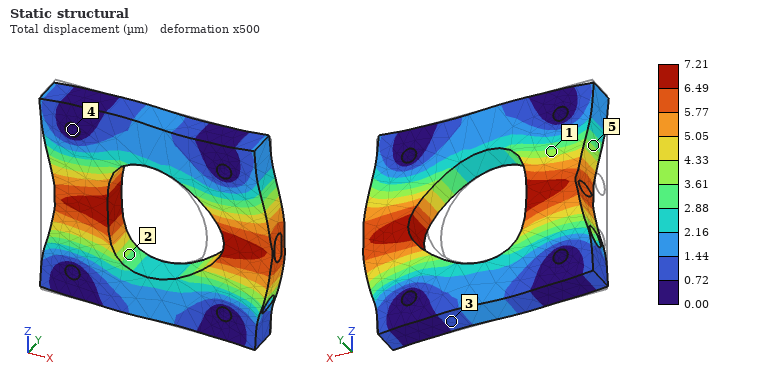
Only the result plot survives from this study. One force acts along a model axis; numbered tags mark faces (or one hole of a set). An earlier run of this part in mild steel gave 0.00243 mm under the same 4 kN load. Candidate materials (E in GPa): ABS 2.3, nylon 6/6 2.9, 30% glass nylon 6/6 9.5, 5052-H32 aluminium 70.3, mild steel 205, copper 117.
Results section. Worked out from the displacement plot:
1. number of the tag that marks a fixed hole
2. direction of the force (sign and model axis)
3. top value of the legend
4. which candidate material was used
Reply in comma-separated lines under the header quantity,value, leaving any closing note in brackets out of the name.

quantity,value
number of the tag that marks a fixed hole,4
direction of the force,+X
top value of the legend,7.21 µm
which candidate material was used,5052-H32 aluminium
